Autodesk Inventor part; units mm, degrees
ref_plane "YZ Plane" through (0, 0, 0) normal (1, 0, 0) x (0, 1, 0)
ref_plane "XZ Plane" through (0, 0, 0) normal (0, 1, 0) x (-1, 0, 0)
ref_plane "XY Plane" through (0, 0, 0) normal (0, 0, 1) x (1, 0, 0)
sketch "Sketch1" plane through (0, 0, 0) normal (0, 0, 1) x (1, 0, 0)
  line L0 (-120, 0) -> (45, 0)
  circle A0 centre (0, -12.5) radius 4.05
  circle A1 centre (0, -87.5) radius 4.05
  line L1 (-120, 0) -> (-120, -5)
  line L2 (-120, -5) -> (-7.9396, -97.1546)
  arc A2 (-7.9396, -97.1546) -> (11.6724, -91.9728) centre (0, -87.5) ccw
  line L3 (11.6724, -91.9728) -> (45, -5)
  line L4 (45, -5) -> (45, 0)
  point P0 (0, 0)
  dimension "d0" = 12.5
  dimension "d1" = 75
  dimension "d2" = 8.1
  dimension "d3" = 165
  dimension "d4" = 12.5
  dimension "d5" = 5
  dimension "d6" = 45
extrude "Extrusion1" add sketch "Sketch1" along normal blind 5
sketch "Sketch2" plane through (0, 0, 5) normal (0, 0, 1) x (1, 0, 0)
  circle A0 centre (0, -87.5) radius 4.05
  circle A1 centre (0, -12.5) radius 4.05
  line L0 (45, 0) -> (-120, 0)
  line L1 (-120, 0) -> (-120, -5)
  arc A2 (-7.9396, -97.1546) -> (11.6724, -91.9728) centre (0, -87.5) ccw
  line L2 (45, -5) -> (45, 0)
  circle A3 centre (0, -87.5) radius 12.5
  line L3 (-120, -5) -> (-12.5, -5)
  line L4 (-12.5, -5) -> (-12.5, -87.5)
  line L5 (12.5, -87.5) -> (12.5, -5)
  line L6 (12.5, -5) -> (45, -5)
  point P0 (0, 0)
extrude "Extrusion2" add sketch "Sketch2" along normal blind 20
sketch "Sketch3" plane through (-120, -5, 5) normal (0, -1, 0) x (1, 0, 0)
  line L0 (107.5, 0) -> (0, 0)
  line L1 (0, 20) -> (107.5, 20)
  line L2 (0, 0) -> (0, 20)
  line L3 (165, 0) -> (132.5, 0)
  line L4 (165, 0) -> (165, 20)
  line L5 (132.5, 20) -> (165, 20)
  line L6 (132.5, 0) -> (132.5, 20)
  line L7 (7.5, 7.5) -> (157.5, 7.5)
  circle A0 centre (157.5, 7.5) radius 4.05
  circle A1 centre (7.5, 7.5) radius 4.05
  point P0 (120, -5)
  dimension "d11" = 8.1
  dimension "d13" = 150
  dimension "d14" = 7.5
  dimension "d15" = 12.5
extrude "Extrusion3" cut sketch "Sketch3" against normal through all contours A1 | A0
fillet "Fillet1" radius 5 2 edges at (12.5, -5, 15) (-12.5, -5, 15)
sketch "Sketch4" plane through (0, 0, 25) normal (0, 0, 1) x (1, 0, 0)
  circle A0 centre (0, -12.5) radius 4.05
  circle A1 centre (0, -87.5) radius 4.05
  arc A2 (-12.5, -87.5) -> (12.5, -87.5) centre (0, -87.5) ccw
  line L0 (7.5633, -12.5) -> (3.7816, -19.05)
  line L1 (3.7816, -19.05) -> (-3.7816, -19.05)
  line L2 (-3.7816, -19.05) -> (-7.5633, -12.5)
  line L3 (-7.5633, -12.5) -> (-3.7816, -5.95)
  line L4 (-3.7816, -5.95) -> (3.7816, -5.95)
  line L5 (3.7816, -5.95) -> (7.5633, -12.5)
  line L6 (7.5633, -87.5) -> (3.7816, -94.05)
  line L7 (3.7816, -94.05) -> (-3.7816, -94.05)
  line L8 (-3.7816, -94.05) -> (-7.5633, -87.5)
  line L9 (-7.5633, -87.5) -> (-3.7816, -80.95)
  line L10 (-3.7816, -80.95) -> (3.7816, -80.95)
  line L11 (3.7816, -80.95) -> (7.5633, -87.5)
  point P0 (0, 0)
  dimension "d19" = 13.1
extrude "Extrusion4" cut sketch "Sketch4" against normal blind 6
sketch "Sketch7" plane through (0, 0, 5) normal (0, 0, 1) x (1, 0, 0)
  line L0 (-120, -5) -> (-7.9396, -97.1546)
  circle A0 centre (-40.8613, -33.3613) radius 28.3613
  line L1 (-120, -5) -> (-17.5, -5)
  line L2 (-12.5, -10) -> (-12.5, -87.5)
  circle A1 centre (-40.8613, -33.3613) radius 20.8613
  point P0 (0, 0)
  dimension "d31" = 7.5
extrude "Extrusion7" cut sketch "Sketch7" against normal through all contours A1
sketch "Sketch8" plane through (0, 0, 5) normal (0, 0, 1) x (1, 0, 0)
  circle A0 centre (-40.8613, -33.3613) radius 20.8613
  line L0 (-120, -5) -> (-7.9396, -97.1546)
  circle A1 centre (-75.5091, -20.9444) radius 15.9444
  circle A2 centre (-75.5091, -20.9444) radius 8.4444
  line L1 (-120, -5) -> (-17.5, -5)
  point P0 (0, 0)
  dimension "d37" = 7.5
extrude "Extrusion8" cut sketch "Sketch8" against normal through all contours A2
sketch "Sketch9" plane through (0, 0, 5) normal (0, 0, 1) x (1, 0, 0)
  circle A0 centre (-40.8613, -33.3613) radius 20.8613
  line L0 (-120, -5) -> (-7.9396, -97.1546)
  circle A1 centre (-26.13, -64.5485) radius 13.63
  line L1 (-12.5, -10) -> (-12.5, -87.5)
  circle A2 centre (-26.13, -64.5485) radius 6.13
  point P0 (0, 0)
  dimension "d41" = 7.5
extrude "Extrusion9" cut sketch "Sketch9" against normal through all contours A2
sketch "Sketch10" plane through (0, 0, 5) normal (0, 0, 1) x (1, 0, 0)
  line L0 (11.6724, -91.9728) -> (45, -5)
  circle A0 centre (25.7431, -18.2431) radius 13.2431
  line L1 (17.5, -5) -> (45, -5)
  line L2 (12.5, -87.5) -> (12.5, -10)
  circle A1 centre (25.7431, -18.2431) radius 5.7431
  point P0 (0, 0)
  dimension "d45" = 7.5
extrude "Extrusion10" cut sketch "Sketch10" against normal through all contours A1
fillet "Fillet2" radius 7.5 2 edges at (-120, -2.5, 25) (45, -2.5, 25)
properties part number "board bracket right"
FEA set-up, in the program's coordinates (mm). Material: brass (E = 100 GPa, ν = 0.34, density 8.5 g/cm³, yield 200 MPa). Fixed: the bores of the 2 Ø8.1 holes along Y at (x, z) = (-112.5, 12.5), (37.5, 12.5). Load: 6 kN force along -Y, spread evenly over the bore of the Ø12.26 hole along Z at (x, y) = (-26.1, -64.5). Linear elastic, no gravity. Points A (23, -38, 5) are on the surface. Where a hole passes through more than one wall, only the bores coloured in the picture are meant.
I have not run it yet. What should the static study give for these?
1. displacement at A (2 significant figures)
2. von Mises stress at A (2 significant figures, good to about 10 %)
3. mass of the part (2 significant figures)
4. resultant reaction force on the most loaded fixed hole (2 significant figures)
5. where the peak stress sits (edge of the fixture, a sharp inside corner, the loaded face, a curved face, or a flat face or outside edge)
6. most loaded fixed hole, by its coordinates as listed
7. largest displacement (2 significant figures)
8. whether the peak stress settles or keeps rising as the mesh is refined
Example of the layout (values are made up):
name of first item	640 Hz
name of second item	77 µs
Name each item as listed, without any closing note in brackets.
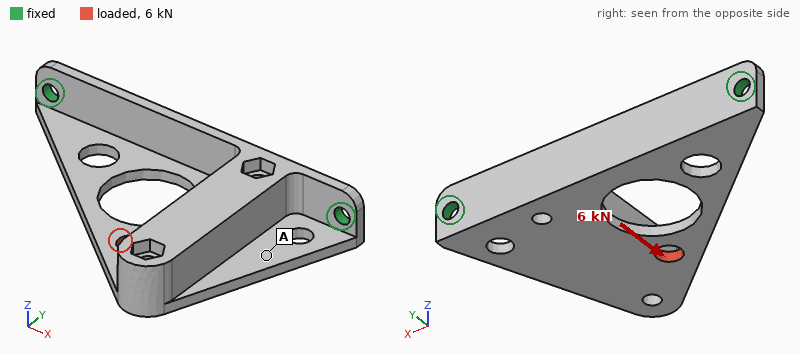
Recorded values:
displacement at A	0.14 mm
von Mises stress at A	20 MPa
mass of the part	810 g
resultant reaction force on the most loaded fixed hole	4.0 kN
where the peak stress sits	edge of the fixture
most loaded fixed hole, by its coordinates as listed	(37.5, 12.5)
largest displacement	0.40 mm
whether the peak stress settles or keeps rising as the mesh is refined	keeps rising
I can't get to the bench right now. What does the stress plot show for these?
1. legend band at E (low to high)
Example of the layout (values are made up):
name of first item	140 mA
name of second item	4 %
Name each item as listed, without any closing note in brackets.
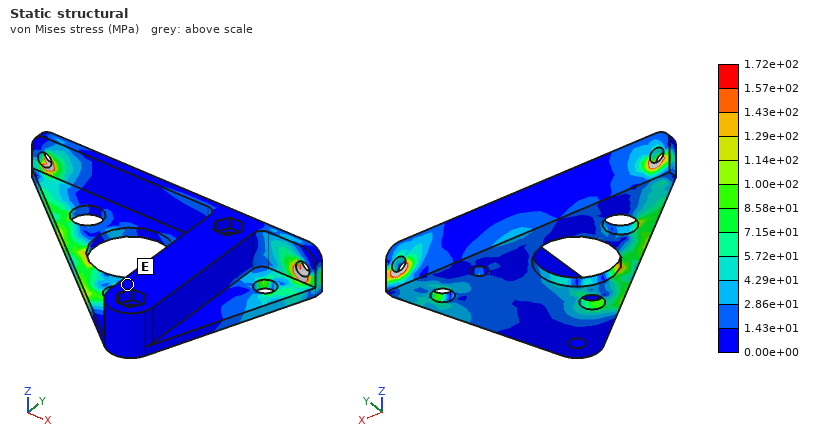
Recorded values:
legend band at E	0.00e+00 to 1.43e+01 MPa
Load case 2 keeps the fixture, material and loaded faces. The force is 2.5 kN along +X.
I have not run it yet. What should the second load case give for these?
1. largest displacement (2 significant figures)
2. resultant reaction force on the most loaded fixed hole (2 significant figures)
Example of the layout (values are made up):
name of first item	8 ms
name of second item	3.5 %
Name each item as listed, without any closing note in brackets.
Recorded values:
largest displacement	67 µm
resultant reaction force on the most loaded fixed hole	1.7 kN
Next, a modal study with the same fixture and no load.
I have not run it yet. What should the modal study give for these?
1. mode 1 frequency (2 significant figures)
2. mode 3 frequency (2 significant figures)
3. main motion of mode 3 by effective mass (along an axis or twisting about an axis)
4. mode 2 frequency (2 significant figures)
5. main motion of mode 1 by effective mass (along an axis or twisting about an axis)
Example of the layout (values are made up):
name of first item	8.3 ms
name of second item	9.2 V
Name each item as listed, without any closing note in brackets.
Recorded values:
mode 1 frequency	260 Hz
mode 3 frequency	1800 Hz
main motion of mode 3 by effective mass	along Y
mode 2 frequency	1400 Hz
main motion of mode 1 by effective mass	along Z
